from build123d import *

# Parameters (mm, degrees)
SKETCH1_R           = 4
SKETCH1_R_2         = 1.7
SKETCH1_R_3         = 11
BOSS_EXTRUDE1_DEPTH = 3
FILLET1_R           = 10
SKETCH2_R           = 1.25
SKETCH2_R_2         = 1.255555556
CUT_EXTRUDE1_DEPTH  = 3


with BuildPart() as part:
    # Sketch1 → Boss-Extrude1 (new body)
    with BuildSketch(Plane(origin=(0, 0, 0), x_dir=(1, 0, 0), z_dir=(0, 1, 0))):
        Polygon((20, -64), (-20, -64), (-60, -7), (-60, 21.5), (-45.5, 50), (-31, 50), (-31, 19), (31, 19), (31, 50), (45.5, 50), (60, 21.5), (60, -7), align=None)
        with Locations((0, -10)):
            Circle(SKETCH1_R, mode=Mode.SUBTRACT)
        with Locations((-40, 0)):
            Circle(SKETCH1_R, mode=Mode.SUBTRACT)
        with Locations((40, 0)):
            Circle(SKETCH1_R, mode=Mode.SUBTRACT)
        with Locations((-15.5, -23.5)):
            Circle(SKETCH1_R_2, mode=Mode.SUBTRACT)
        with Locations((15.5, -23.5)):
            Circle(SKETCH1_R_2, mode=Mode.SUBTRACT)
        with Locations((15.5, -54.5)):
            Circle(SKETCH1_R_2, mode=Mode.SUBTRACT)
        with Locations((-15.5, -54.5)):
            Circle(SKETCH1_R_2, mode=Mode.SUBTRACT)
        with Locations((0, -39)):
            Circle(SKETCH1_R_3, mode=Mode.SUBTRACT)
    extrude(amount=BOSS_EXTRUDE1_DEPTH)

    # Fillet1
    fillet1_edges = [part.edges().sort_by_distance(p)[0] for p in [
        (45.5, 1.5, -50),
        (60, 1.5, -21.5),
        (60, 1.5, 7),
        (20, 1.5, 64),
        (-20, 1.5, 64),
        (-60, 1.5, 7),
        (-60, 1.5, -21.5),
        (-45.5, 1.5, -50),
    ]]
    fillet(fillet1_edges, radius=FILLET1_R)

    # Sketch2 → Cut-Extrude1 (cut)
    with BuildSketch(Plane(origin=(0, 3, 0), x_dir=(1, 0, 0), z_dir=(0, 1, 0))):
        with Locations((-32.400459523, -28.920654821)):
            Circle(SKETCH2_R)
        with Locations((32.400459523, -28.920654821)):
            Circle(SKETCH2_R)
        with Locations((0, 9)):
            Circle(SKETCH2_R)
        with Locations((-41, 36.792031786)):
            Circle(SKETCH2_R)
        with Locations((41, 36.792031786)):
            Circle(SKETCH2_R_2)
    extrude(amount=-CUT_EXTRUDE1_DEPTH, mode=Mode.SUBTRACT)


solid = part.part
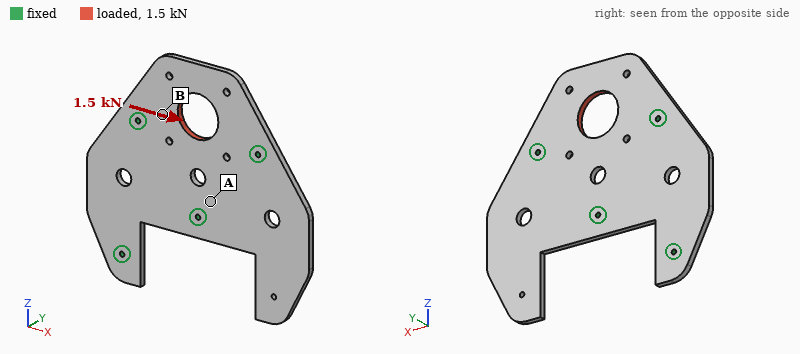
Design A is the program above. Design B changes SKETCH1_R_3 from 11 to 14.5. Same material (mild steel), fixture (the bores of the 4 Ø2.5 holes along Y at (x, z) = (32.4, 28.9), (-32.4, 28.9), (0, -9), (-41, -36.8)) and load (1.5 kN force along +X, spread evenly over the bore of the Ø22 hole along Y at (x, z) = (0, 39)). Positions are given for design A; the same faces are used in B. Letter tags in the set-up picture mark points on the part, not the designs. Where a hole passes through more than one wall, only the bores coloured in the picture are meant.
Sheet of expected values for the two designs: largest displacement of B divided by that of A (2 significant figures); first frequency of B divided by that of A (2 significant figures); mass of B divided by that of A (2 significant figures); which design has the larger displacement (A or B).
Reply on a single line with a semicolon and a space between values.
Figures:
1.3; 1.00; 0.97; B
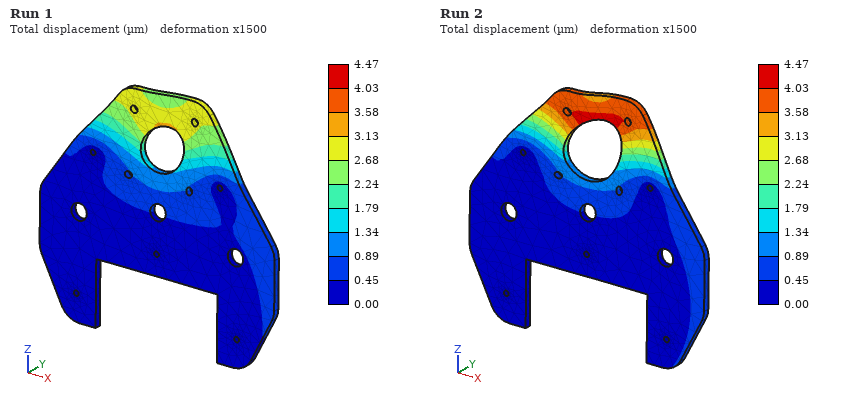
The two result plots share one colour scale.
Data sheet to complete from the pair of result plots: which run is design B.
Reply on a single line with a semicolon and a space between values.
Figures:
Run 2
